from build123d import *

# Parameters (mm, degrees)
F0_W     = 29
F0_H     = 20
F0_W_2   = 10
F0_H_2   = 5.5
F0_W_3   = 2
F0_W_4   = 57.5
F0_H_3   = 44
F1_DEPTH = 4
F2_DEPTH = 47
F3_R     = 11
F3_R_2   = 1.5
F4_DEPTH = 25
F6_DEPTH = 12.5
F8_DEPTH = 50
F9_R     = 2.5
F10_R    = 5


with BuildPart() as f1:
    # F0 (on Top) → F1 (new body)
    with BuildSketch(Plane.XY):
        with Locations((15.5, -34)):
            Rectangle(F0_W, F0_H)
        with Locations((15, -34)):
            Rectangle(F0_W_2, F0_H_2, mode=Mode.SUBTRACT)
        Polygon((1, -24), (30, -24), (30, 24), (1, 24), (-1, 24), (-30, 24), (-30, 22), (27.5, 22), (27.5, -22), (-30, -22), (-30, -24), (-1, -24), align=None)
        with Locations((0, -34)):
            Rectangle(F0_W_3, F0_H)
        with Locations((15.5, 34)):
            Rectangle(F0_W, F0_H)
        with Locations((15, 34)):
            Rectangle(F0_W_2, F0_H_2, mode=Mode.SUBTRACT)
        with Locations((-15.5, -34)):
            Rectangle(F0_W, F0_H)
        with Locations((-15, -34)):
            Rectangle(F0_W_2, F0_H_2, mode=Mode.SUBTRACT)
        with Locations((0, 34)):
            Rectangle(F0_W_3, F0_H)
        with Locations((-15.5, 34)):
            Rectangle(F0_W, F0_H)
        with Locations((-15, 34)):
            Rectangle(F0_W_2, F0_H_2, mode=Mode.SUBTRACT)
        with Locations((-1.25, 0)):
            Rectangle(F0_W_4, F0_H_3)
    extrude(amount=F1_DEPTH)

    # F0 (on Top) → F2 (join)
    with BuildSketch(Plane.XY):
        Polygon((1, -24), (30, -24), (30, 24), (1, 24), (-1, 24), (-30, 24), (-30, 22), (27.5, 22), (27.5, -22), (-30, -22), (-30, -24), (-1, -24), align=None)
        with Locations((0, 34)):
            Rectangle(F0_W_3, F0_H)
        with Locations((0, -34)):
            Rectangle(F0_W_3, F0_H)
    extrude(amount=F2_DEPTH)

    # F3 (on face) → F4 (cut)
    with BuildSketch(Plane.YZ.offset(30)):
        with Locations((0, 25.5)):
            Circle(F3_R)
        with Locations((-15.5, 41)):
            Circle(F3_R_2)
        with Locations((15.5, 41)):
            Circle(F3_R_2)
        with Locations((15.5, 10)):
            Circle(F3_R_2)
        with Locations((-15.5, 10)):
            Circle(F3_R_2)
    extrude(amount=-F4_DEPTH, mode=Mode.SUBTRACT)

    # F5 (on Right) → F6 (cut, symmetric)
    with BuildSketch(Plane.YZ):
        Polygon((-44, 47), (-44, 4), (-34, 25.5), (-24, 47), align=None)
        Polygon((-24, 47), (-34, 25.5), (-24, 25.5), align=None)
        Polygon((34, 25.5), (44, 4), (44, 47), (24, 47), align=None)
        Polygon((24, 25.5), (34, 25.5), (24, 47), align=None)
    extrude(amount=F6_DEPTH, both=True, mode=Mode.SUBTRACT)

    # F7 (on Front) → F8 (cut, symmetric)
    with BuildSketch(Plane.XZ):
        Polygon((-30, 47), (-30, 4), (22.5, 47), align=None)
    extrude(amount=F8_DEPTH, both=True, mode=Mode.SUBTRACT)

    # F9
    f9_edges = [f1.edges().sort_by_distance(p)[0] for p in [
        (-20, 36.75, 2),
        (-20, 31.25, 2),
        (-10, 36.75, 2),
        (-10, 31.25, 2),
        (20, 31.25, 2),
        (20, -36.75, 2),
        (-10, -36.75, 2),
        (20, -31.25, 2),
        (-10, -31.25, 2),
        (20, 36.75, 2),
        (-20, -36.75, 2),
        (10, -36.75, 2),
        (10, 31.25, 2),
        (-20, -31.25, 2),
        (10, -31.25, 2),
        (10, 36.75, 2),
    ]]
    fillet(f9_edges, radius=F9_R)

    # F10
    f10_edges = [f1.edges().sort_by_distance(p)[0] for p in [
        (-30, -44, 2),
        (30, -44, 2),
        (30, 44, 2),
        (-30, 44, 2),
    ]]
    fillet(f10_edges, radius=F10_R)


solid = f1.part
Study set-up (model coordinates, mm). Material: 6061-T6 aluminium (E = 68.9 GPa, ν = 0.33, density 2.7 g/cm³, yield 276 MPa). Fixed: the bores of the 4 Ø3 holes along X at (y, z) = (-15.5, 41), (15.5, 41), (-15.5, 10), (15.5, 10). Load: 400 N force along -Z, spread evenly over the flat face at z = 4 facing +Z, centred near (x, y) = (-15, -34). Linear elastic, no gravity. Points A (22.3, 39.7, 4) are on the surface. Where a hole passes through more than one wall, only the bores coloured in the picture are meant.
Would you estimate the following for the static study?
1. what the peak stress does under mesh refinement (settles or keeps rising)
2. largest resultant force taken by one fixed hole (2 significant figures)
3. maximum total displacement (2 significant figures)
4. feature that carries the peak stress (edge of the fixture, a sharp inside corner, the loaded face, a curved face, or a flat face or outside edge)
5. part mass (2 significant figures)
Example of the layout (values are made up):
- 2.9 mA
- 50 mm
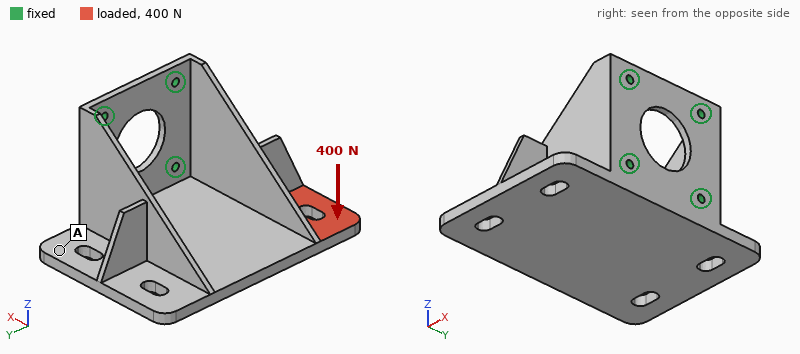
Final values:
- keeps rising
- 640 N
- 0.26 mm
- edge of the fixture
- 84 g
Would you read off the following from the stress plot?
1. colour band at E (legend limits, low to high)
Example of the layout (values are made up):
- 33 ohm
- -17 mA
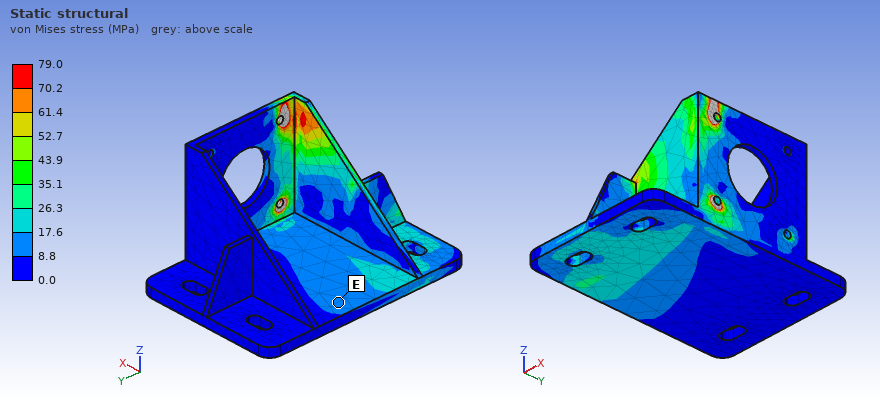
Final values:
- 8.8 to 17.6 MPa
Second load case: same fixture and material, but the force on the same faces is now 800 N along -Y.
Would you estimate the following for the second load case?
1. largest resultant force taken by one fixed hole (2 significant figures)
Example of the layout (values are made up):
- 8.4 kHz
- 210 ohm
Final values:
- 1.2 kN
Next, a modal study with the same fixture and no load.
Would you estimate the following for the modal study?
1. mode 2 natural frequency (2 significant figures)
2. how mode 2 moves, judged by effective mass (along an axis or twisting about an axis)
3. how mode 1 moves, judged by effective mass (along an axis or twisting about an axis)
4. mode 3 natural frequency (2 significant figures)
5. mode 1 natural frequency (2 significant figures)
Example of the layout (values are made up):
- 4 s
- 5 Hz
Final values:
- 2200 Hz
- along Z
- along Y
- 3200 Hz
- 1600 Hz
